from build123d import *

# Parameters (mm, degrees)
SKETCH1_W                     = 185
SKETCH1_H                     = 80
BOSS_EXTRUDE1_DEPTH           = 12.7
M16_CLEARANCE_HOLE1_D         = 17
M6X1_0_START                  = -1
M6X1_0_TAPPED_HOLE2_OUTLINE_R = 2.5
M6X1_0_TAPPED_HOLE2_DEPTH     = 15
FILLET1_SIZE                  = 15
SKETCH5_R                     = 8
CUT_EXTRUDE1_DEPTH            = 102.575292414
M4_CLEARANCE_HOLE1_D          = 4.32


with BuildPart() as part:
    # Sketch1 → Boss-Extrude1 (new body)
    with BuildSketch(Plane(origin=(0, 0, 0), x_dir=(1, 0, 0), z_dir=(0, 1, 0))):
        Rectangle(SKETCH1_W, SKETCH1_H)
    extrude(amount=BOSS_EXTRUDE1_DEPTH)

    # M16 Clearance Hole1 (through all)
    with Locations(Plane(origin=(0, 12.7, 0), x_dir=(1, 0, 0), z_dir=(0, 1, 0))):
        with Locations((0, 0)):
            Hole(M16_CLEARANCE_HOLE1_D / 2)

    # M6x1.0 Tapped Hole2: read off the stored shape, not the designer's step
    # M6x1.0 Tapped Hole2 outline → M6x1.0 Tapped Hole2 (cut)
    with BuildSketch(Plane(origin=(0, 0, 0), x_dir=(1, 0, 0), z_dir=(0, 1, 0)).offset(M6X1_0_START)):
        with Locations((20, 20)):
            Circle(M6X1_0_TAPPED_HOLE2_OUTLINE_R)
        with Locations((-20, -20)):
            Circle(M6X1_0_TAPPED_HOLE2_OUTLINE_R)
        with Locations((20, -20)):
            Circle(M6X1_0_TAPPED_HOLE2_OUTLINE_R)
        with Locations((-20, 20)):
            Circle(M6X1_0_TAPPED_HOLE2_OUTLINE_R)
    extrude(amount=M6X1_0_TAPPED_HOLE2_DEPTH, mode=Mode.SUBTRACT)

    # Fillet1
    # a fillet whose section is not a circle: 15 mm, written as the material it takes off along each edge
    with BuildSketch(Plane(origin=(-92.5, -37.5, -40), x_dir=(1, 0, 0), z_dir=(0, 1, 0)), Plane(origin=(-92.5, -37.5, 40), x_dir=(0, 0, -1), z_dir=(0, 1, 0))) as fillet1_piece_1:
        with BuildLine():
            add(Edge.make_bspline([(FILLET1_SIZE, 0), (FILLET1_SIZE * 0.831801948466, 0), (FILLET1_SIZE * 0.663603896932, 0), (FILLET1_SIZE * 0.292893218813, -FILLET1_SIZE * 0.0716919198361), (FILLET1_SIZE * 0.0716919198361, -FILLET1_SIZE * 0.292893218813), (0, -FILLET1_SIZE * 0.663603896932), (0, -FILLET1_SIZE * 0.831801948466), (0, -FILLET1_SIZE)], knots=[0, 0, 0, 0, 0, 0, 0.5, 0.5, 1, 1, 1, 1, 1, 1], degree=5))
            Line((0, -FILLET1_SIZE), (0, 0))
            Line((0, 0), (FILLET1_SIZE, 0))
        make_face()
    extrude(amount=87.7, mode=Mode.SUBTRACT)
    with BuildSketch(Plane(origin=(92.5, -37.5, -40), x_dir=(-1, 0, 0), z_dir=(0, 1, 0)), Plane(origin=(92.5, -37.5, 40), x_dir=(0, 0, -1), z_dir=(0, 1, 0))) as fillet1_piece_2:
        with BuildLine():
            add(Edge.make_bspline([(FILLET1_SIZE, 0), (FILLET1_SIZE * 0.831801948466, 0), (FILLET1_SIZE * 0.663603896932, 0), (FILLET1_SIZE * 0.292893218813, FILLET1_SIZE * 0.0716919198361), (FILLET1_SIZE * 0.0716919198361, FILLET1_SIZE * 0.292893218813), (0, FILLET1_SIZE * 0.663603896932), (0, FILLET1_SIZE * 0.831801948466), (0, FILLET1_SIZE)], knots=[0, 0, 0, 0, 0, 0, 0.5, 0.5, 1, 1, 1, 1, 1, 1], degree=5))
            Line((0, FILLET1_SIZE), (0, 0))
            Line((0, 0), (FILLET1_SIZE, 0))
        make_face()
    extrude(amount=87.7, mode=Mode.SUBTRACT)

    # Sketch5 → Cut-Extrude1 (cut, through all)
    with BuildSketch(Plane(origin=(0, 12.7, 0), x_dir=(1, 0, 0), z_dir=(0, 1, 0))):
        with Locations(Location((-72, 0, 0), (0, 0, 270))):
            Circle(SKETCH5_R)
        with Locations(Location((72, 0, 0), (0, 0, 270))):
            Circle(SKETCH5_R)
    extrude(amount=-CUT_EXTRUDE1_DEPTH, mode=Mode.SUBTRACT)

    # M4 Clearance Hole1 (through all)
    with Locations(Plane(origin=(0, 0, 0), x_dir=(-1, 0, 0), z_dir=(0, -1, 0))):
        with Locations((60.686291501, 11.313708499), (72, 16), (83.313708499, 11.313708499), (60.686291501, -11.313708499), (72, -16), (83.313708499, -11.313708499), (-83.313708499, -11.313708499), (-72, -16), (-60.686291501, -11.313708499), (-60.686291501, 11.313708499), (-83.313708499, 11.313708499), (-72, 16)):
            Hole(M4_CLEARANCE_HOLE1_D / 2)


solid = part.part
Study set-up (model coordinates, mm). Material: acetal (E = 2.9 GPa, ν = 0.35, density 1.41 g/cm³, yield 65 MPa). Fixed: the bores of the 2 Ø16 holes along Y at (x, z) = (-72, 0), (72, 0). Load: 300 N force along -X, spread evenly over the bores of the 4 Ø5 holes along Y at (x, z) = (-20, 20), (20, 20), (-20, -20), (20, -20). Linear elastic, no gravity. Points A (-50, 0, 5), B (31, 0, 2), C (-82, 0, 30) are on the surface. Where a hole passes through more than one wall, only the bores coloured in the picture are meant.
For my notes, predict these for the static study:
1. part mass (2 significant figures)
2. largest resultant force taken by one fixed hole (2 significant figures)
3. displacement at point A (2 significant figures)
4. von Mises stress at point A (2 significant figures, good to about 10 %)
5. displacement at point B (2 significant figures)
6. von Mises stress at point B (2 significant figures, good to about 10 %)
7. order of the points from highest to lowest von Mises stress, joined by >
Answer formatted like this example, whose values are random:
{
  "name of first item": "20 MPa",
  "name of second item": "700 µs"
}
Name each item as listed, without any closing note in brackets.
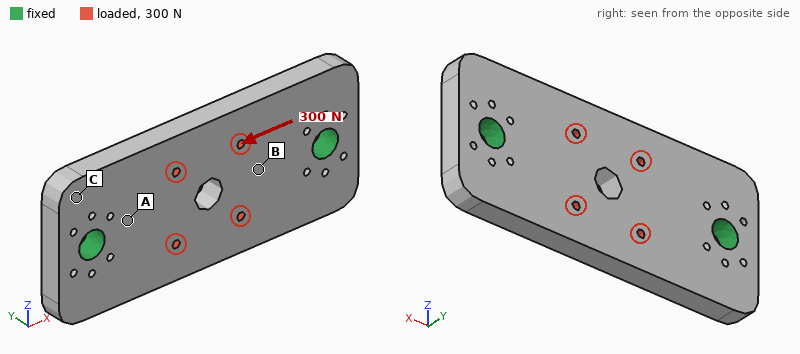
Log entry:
{
  "part mass": "250 g",
  "largest resultant force taken by one fixed hole": "150 N",
  "displacement at point A": "1.8 µm",
  "von Mises stress at point A": "0.29 MPa",
  "displacement at point B": "3.2 µm",
  "von Mises stress at point B": "0.15 MPa",
  "order of the points from highest to lowest von Mises stress, joined by >": "A > B > C"
}
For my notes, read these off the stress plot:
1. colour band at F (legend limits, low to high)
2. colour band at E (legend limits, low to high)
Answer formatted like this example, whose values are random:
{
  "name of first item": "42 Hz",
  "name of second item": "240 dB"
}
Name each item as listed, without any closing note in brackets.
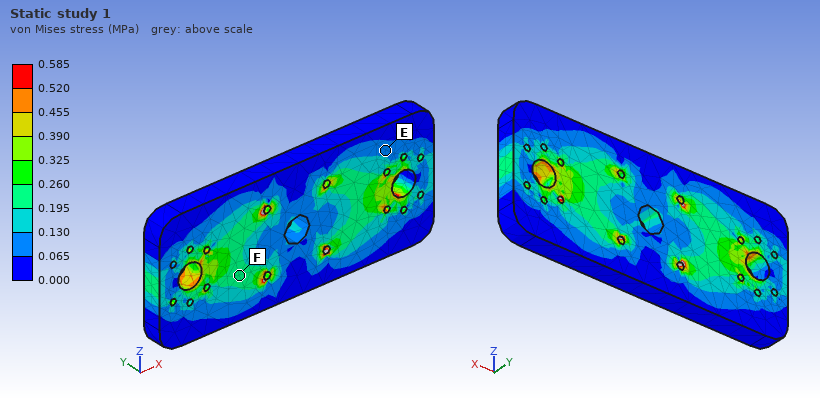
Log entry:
{
  "colour band at F": "0.195 to 0.260 MPa",
  "colour band at E": "0.065 to 0.130 MPa"
}
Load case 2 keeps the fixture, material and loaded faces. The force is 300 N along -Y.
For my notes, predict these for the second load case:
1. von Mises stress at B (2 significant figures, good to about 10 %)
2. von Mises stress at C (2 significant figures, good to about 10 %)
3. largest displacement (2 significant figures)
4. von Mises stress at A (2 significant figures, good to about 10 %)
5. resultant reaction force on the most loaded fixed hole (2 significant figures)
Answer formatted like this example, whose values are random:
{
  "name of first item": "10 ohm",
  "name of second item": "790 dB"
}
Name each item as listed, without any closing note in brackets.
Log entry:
{
  "von Mises stress at B": "0.67 MPa",
  "von Mises stress at C": "0.47 MPa",
  "largest displacement": "0.12 mm",
  "von Mises stress at A": "1.1 MPa",
  "resultant reaction force on the most loaded fixed hole": "150 N"
}
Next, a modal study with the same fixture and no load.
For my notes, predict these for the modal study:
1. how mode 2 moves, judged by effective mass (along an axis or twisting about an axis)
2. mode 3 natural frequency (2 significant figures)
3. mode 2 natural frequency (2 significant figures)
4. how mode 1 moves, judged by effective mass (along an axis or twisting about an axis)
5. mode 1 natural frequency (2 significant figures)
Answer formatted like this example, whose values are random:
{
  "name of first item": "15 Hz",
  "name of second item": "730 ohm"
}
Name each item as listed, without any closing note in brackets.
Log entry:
{
  "how mode 2 moves, judged by effective mass": "twisting about X",
  "mode 3 natural frequency": "1800 Hz",
  "mode 2 natural frequency": "920 Hz",
  "how mode 1 moves, judged by effective mass": "along Y",
  "mode 1 natural frequency": "820 Hz"
}
